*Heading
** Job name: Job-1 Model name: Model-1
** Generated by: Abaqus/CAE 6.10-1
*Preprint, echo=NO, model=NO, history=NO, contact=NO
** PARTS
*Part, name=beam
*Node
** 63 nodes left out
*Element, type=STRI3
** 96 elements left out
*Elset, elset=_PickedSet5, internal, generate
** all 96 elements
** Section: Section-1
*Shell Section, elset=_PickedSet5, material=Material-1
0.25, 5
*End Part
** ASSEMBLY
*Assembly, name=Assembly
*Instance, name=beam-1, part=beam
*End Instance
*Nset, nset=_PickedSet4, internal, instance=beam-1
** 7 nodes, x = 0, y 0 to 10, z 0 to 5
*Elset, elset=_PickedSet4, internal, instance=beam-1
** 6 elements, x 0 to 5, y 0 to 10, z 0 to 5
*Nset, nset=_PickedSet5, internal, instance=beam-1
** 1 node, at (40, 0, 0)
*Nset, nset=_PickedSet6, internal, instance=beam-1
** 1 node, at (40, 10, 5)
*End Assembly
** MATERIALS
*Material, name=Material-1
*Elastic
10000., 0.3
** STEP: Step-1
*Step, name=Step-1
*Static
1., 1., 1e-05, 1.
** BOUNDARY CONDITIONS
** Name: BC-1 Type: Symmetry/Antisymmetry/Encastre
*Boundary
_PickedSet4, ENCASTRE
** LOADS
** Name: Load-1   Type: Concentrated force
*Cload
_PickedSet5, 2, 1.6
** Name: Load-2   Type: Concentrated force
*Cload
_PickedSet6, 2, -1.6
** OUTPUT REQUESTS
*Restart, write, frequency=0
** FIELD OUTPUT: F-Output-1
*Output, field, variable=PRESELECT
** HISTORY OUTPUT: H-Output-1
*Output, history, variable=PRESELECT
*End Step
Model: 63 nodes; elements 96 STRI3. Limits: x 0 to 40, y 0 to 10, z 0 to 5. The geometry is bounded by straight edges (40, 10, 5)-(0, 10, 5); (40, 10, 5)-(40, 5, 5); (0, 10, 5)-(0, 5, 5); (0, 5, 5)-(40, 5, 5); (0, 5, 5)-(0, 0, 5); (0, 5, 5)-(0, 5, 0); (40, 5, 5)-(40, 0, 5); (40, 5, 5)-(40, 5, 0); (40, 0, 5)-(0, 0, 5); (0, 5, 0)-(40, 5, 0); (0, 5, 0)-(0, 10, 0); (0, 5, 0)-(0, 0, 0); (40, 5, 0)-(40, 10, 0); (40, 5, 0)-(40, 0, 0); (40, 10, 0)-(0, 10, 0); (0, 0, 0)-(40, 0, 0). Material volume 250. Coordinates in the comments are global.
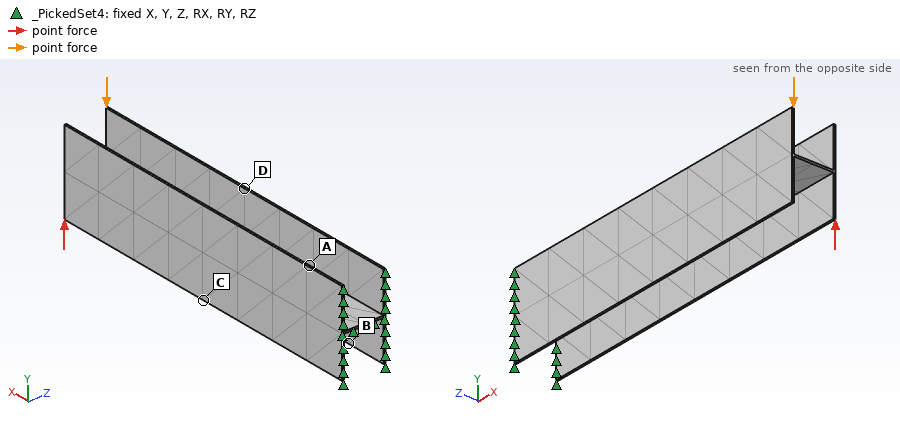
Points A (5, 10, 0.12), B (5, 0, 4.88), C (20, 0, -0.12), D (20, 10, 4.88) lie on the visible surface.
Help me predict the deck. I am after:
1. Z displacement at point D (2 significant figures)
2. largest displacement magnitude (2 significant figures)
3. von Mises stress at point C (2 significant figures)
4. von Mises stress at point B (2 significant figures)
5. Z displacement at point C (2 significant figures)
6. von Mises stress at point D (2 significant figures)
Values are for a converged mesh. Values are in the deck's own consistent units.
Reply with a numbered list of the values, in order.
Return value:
1. 0.10
2. 0.31
3. 7.2
4. 13
5. -0.10
6. 7.5
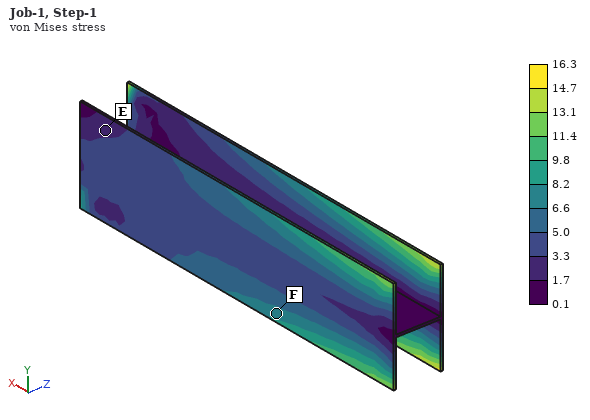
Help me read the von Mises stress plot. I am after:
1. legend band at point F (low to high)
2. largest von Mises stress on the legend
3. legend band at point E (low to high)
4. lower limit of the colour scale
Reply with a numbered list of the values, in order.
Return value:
1. 6.6 to 8.2
2. 16.3
3. 1.7 to 3.3
4. 0.1
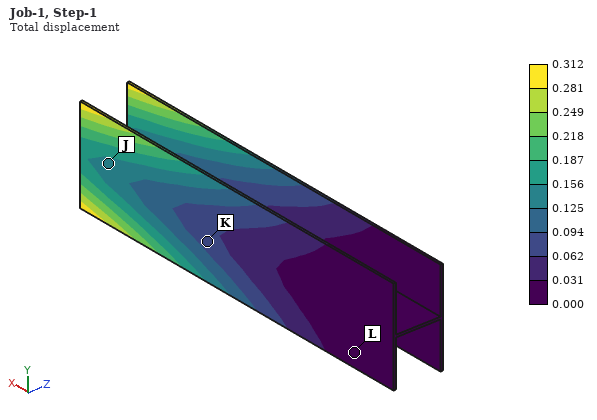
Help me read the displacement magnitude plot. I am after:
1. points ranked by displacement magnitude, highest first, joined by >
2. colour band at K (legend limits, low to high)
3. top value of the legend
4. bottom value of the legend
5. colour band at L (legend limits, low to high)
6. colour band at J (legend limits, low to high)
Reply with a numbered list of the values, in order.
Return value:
1. J > K > L
2. 0.062 to 0.094
3. 0.312
4. 0.000
5. 0.000 to 0.031
6. 0.125 to 0.156
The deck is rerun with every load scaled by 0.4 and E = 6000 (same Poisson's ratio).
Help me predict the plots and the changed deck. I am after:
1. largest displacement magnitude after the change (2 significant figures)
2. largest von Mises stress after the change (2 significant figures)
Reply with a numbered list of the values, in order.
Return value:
1. 0.21
2. 6.5
